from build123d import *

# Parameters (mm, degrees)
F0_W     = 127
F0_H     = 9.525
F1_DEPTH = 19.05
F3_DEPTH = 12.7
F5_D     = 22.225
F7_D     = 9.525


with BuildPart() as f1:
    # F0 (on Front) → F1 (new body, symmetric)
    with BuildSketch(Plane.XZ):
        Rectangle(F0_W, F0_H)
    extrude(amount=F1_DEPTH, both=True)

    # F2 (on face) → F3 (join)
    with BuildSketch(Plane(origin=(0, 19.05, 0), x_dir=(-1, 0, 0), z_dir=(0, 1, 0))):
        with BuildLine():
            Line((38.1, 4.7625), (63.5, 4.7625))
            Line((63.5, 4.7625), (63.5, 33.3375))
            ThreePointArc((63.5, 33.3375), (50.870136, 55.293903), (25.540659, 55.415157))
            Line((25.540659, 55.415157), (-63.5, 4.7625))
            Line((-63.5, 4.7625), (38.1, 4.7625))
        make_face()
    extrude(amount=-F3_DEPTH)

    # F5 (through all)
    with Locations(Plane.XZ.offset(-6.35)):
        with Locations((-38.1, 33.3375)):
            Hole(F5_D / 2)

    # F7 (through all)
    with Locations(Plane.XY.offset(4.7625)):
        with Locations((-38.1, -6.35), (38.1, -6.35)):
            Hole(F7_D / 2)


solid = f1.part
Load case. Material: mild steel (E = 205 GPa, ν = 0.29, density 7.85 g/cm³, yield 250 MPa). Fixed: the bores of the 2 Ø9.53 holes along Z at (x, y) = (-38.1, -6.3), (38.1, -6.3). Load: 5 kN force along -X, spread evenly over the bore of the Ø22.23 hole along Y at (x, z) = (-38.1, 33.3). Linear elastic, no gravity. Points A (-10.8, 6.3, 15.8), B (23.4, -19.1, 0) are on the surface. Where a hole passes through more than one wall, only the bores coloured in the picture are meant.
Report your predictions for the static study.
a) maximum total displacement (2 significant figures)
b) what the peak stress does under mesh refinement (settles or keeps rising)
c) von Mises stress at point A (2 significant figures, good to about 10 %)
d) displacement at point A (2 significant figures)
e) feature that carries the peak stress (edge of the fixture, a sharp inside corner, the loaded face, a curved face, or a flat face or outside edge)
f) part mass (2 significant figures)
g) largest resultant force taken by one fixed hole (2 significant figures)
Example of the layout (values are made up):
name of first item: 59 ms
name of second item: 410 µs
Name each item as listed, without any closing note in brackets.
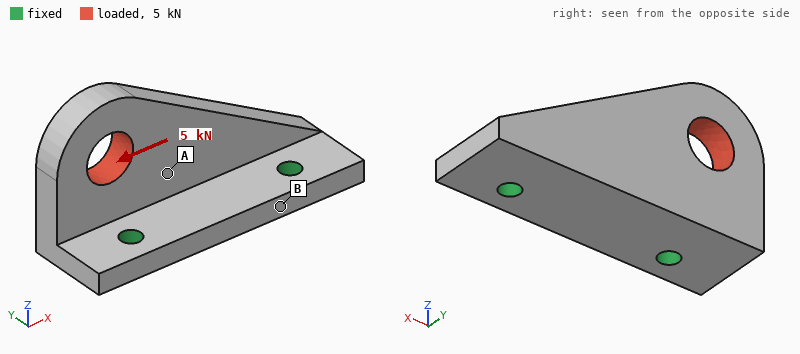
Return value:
maximum total displacement: 19 µm
what the peak stress does under mesh refinement: keeps rising
von Mises stress at point A: 13 MPa
displacement at point A: 4.6 µm
feature that carries the peak stress: edge of the fixture
part mass: 730 g
largest resultant force taken by one fixed hole: 3.4 kN
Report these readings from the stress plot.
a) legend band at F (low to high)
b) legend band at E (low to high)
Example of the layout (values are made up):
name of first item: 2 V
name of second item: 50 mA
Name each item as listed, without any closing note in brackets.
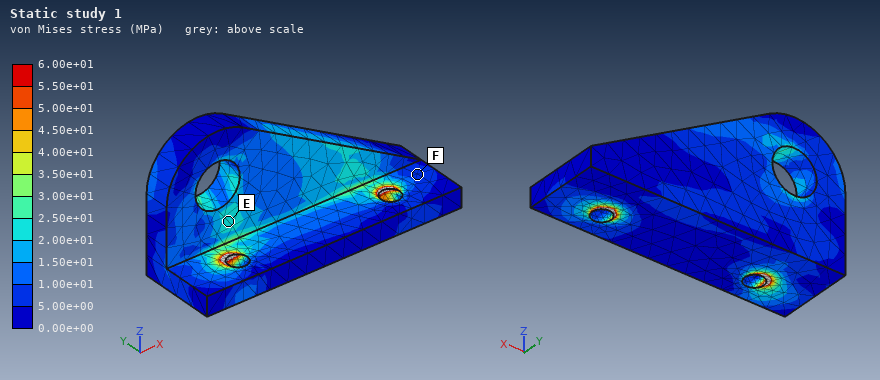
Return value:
legend band at F: 5.00e+00 to 1.00e+01 MPa
legend band at E: 2.00e+01 to 2.50e+01 MPa
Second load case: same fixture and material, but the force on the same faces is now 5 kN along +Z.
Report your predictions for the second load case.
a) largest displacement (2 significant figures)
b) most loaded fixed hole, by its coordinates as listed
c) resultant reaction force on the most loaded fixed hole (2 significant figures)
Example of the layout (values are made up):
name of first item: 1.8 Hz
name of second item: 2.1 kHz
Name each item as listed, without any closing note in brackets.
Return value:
largest displacement: 55 µm
most loaded fixed hole, by its coordinates as listed: (-38.1, -6.3)
resultant reaction force on the most loaded fixed hole: 4.8 kN
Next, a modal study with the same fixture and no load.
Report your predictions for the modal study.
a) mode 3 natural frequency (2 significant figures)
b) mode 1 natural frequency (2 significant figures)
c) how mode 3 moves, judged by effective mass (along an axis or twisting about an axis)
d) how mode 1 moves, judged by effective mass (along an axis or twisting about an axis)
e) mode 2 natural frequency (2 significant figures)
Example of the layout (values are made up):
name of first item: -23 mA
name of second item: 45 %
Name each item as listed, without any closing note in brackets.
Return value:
mode 3 natural frequency: 6300 Hz
mode 1 natural frequency: 2100 Hz
how mode 3 moves, judged by effective mass: along Z
how mode 1 moves, judged by effective mass: along Y
mode 2 natural frequency: 5000 Hz
